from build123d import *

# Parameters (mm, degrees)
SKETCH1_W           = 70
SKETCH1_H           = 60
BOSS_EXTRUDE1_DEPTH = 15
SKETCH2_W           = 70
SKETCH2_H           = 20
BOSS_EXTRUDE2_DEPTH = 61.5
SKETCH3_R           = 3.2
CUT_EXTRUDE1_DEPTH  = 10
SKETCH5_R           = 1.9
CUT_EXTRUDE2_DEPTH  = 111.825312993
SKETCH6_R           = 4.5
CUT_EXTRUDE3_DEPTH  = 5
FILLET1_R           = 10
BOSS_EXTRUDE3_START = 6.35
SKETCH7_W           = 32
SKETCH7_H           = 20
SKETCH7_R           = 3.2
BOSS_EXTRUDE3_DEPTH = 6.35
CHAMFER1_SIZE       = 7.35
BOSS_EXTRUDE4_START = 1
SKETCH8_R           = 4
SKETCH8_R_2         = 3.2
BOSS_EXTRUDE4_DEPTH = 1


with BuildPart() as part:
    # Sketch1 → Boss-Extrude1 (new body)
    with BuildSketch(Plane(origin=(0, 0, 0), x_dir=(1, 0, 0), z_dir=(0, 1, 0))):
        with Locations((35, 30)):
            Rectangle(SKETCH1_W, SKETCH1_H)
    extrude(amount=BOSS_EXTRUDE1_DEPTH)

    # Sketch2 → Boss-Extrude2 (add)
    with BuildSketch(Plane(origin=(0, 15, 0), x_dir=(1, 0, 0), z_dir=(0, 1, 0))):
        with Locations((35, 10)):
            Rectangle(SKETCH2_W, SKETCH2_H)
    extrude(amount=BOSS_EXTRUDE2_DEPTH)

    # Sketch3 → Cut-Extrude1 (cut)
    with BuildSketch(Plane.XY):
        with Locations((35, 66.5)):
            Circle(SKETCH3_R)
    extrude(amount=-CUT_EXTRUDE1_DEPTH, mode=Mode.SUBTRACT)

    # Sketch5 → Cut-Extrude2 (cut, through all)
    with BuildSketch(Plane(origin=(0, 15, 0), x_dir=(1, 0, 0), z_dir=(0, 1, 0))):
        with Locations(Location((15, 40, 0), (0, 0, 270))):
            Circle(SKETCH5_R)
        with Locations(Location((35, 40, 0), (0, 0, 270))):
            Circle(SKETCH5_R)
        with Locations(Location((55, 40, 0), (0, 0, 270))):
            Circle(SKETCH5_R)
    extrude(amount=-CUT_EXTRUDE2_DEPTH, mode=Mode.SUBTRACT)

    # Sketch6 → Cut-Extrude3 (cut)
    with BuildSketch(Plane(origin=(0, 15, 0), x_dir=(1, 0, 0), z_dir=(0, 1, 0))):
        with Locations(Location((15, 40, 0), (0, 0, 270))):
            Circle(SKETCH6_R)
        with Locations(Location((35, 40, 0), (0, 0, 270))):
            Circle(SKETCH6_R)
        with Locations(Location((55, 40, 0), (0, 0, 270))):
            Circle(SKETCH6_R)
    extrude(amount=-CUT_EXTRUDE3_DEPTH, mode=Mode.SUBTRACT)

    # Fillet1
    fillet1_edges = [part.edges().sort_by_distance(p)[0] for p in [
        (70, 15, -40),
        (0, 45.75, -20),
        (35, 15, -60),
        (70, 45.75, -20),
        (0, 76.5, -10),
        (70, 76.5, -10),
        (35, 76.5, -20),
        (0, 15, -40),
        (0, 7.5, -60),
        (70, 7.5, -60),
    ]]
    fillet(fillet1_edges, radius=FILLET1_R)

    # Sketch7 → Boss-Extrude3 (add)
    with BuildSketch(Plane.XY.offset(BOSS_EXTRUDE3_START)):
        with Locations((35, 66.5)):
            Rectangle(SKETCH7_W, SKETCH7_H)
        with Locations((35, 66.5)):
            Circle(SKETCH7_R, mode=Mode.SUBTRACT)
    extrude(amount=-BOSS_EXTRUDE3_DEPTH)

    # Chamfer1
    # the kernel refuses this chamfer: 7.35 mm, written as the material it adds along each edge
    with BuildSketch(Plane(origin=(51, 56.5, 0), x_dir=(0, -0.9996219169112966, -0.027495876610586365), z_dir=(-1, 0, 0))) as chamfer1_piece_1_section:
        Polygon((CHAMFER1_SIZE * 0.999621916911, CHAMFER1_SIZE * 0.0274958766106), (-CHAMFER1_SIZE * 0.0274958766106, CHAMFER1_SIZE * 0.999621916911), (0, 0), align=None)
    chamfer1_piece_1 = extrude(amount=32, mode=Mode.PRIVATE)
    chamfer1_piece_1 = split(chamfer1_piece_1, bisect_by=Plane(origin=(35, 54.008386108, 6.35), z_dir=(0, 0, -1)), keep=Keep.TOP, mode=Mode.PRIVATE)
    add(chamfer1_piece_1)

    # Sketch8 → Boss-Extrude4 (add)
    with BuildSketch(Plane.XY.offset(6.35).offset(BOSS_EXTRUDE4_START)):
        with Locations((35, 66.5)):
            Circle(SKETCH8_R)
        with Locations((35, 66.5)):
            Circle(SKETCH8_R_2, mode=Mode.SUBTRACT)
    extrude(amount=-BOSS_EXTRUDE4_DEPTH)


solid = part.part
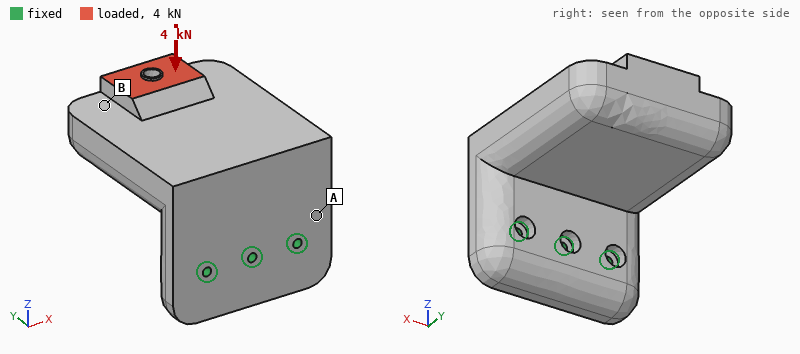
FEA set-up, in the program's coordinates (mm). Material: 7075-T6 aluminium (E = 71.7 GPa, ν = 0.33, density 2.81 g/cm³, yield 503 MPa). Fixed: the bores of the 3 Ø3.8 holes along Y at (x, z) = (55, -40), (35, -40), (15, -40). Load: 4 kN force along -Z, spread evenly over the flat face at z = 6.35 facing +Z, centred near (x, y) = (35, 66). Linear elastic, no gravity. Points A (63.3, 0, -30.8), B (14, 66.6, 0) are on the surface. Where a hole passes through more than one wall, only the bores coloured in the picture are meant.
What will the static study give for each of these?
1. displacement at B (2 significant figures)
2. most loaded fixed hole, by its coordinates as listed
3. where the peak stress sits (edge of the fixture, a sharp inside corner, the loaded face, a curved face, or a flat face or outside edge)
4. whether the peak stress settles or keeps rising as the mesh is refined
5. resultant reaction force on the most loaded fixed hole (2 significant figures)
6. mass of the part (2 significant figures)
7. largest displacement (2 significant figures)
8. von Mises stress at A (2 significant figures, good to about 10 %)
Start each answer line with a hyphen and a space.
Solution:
- 0.58 mm
- (35, -40)
- edge of the fixture
- keeps rising
- 1.9 kN
- 400 g
- 0.69 mm
- 85 MPa
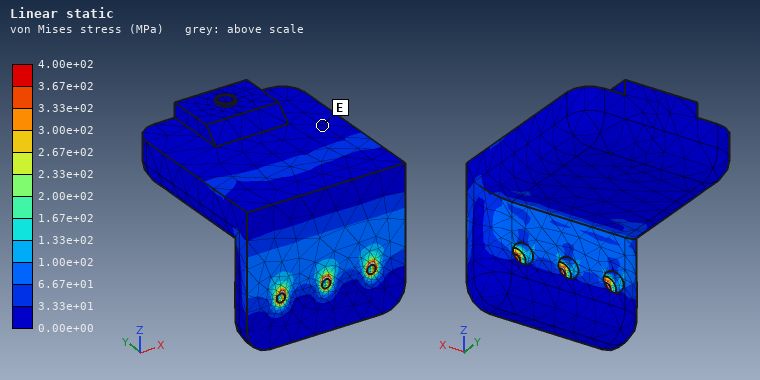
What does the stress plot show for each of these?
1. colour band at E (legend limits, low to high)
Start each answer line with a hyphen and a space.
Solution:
- 0.00e+00 to 3.33e+01 MPa
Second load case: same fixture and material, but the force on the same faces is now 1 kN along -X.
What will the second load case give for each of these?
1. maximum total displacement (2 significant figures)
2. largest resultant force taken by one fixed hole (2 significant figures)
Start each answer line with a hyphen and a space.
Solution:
- 38 µm
- 1.8 kN
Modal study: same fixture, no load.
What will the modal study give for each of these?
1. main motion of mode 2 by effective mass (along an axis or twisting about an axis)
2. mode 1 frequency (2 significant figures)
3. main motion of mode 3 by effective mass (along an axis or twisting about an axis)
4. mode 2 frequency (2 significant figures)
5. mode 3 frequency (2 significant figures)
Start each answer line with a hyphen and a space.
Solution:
- along X
- 1100 Hz
- along Y
- 2200 Hz
- 4700 Hz
